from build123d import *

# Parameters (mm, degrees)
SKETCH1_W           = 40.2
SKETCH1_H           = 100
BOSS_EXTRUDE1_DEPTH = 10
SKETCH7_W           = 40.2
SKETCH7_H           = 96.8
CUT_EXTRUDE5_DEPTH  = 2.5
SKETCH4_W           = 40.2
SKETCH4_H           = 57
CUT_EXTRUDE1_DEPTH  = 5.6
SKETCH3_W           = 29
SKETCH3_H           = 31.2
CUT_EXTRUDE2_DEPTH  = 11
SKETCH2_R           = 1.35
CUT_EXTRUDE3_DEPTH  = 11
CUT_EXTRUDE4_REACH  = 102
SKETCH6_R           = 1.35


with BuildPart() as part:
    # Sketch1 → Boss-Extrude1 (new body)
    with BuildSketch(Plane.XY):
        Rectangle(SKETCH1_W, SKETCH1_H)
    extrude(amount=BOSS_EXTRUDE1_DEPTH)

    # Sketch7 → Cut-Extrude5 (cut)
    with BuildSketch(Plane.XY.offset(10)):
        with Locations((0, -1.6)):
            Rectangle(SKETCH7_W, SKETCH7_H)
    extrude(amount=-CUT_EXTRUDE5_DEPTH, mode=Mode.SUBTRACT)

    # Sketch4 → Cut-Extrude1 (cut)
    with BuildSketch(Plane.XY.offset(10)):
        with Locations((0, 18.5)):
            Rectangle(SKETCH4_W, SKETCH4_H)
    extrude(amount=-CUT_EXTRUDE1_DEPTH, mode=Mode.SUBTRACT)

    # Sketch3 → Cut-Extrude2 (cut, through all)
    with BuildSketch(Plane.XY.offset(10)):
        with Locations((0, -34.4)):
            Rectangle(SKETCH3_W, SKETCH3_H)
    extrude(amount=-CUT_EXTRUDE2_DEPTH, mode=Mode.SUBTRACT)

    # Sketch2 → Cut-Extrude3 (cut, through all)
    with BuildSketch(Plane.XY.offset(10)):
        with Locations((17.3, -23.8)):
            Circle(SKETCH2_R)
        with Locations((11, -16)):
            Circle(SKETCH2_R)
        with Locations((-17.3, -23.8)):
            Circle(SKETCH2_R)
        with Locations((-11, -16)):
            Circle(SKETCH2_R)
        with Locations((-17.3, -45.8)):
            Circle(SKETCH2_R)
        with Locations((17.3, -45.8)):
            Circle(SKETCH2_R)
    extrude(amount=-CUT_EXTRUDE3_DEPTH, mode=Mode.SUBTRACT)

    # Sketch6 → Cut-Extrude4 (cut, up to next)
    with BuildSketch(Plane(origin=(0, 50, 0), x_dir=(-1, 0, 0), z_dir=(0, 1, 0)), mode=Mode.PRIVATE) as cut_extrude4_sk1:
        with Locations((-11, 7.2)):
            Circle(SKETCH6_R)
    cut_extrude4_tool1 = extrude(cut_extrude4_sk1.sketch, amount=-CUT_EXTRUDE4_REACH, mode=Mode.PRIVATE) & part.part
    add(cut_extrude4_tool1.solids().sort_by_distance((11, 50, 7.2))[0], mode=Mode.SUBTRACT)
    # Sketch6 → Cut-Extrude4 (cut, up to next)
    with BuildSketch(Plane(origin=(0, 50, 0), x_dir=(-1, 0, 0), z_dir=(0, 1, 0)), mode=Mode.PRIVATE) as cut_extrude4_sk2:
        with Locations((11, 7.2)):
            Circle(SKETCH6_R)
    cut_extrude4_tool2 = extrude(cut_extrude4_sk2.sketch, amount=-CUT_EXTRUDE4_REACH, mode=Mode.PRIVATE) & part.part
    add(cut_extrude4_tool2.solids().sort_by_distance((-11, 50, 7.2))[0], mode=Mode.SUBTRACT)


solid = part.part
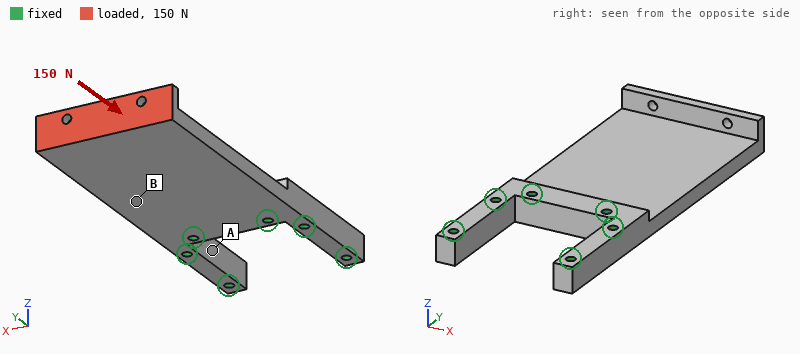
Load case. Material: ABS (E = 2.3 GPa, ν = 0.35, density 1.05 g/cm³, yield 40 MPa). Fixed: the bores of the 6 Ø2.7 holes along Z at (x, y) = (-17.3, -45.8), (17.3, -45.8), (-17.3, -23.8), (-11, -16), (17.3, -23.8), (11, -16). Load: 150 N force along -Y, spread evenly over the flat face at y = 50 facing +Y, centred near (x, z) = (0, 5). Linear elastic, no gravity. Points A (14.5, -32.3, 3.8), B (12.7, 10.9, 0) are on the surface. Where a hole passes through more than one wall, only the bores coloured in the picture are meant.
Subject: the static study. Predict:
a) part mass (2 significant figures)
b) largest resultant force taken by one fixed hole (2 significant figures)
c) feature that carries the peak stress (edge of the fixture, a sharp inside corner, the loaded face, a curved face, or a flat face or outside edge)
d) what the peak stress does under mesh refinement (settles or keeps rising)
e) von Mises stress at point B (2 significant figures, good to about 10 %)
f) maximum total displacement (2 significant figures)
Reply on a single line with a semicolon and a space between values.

17 g; 59 N; edge of the fixture; keeps rising; 2.2 MPa; 1.2 mm
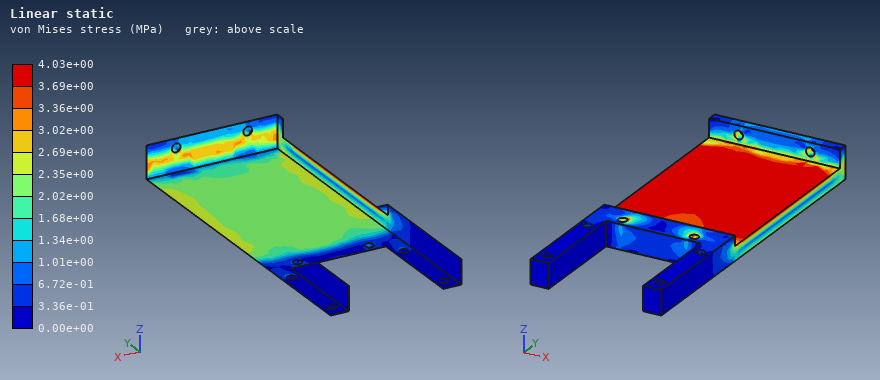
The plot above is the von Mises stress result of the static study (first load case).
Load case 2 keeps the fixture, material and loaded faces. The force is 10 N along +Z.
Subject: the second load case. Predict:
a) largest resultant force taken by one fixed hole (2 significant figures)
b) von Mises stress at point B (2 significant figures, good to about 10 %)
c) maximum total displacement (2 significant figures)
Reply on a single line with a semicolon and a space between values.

13 N; 2.9 MPa; 1.3 mm
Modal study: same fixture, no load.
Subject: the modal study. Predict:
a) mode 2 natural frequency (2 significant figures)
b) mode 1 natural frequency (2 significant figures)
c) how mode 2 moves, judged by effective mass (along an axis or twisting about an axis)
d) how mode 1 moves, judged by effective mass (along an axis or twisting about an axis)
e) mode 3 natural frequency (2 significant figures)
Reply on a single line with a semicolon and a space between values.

820 Hz; 240 Hz; twisting about Y; along Z; 1500 Hz
